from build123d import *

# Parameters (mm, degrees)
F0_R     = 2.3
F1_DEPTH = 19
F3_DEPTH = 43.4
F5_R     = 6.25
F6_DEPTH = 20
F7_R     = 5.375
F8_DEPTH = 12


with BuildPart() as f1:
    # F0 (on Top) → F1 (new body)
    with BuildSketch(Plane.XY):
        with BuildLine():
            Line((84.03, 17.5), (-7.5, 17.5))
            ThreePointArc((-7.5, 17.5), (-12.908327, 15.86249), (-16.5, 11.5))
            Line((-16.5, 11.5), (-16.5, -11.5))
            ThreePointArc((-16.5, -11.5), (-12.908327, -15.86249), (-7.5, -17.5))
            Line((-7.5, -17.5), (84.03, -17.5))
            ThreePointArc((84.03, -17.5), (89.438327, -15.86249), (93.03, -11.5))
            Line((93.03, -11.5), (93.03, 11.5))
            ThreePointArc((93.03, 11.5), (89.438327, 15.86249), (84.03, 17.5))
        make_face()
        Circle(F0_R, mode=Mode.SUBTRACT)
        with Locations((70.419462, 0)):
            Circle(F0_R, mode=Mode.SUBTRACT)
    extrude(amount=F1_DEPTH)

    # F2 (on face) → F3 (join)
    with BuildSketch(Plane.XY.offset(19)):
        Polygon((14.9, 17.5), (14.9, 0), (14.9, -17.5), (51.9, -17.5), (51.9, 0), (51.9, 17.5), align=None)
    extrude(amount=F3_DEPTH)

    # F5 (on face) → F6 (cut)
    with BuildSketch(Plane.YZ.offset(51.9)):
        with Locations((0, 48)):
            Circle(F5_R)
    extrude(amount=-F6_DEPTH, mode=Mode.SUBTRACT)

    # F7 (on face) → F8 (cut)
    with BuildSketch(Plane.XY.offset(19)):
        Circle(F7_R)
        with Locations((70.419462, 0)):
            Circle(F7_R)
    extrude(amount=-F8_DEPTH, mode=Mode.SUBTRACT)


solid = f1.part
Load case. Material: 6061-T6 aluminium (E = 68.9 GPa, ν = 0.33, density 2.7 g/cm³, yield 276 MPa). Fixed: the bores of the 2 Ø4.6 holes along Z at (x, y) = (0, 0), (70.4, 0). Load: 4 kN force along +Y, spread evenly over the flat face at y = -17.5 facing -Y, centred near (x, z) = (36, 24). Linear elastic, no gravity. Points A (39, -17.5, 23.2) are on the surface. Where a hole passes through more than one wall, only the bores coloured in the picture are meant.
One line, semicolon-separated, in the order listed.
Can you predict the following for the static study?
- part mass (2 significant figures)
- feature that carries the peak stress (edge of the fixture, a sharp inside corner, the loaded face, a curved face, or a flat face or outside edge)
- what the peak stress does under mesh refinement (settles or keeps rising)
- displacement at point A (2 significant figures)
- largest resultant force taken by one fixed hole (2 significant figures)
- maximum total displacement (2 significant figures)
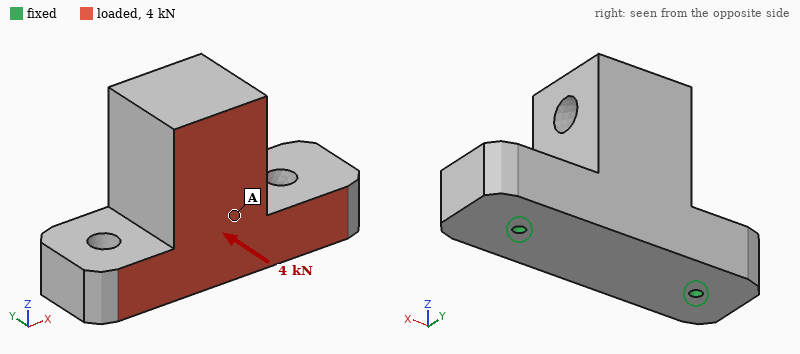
330 g; edge of the fixture; keeps rising; 0.097 mm; 2.0 kN; 0.22 mm
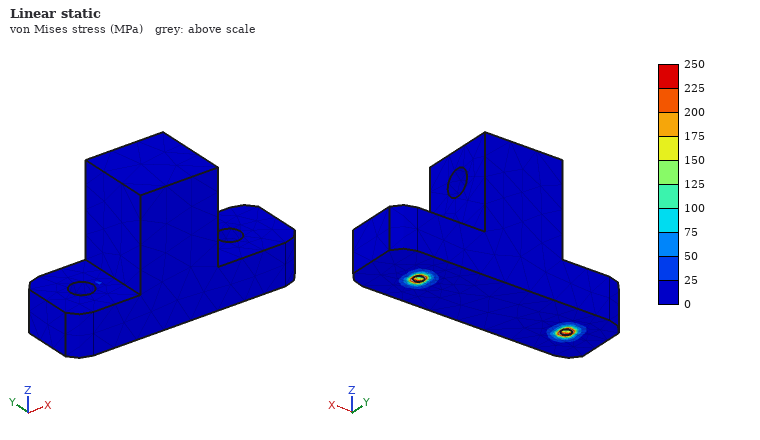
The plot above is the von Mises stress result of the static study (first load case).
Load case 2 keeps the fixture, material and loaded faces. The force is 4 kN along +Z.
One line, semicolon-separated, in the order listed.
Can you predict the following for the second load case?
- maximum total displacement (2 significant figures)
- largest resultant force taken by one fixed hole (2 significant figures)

0.18 mm; 2.3 kN
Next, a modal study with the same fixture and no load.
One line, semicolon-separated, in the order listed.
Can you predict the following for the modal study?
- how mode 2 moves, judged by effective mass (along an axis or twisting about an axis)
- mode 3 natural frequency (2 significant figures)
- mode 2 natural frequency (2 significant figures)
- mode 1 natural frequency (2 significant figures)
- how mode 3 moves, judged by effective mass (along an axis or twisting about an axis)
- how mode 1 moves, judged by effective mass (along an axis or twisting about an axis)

along X; 6500 Hz; 6000 Hz; 1500 Hz; along Z; along Y
